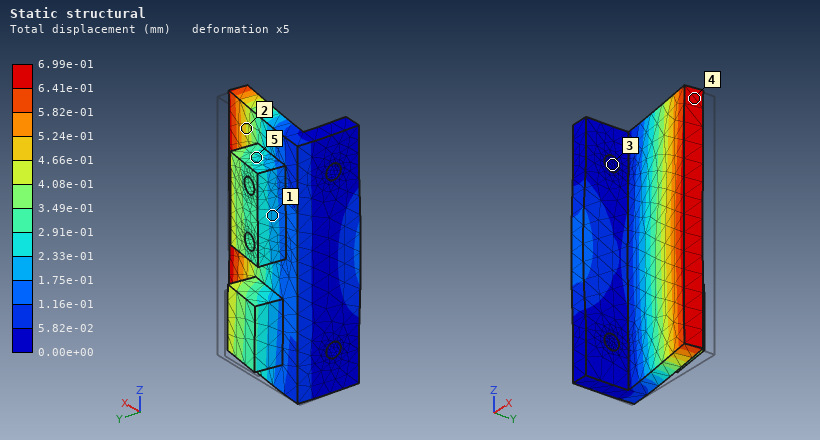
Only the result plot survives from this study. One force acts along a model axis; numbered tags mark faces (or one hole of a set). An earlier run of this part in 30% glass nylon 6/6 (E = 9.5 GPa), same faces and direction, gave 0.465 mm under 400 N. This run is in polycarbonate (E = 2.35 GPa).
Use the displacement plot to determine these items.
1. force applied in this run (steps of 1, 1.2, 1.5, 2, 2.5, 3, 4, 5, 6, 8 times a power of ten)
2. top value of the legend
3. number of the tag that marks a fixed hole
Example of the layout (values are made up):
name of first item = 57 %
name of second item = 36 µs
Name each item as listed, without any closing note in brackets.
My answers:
force applied in this run = 150 N
top value of the legend = 6.99e-01 mm
number of the tag that marks a fixed hole = 3
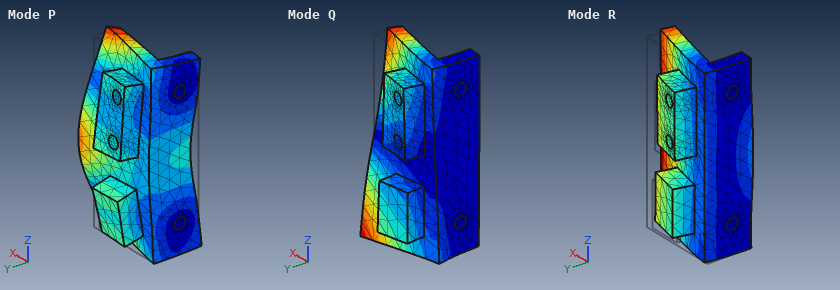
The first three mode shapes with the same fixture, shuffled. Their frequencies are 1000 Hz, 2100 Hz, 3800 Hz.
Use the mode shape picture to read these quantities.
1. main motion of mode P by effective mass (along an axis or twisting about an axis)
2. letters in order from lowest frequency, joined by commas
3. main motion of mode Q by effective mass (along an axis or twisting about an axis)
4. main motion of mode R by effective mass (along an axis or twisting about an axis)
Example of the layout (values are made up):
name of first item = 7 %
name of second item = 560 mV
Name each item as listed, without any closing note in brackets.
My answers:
main motion of mode P by effective mass = along X
letters in order from lowest frequency, joined by commas = R, Q, P
main motion of mode Q by effective mass = twisting about X
main motion of mode R by effective mass = along Y
